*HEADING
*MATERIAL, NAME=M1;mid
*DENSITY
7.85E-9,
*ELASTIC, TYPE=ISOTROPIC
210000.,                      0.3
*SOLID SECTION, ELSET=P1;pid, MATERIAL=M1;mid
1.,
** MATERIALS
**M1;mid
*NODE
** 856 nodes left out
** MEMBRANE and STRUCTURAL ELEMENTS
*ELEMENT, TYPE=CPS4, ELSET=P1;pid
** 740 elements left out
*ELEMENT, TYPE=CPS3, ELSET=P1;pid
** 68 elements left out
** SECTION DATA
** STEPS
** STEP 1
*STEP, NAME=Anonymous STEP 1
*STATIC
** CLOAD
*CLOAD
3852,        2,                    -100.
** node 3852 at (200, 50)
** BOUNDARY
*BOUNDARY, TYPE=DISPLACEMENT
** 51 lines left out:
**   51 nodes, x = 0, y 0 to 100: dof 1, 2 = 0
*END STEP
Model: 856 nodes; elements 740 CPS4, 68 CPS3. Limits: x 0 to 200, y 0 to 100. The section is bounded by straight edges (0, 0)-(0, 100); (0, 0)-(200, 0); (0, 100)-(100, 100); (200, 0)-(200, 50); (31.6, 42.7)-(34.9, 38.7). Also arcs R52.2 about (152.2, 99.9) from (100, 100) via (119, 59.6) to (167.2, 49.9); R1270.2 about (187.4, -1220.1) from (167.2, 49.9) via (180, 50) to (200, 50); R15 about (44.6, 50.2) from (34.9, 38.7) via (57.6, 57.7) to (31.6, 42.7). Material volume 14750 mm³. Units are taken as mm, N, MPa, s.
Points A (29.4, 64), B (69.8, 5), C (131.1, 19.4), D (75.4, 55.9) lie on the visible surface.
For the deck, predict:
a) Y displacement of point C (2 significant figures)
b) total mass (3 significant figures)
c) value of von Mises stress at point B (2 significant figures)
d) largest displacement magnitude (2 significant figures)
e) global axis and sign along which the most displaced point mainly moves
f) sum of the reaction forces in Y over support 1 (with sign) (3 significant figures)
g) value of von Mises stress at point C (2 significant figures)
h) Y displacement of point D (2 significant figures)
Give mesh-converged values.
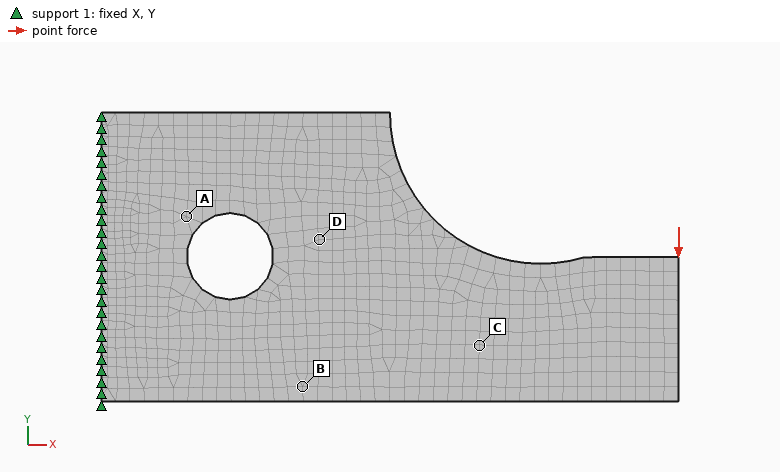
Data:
-0.012 mm
0.116 kg
8.4 MPa
0.037 mm
-Y
100 N
5.0 MPa
-0.0045 mm
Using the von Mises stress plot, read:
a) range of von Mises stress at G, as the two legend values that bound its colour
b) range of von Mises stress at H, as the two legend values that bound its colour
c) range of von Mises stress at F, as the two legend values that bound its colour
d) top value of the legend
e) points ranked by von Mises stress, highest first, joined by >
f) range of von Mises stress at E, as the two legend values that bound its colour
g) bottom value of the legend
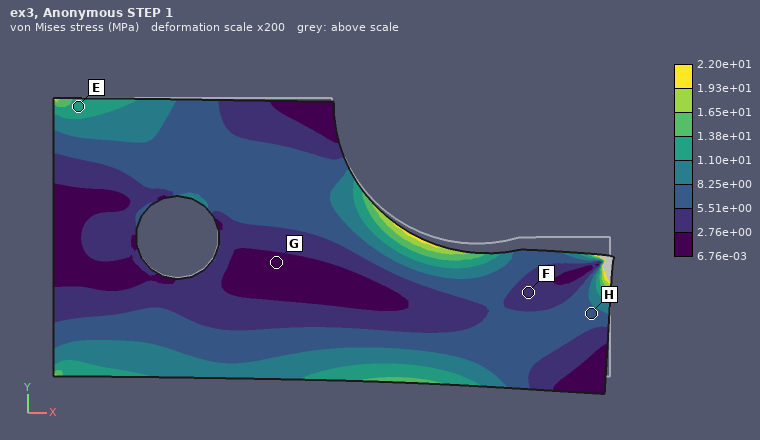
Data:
6.76e-03 to 2.76e+00 MPa
5.51e+00 to 8.25e+00 MPa
2.76e+00 to 5.51e+00 MPa
2.20e+01 MPa
E > H > F > G
1.10e+01 to 1.38e+01 MPa
6.76e-03 MPa
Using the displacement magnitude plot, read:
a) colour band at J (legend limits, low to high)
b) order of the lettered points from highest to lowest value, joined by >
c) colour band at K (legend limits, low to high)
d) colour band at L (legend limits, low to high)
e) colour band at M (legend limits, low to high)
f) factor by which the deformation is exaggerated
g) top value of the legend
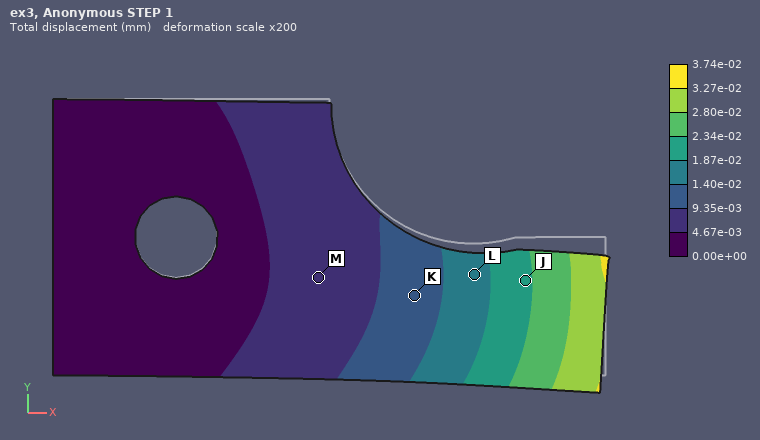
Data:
1.87e-02 to 2.34e-02 mm
J > L > K > M
9.35e-03 to 1.40e-02 mm
1.40e-02 to 1.87e-02 mm
4.67e-03 to 9.35e-03 mm
200
3.74e-02 mm
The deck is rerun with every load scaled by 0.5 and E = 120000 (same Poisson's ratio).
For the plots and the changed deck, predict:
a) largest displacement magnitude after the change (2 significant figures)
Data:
0.033 mm
